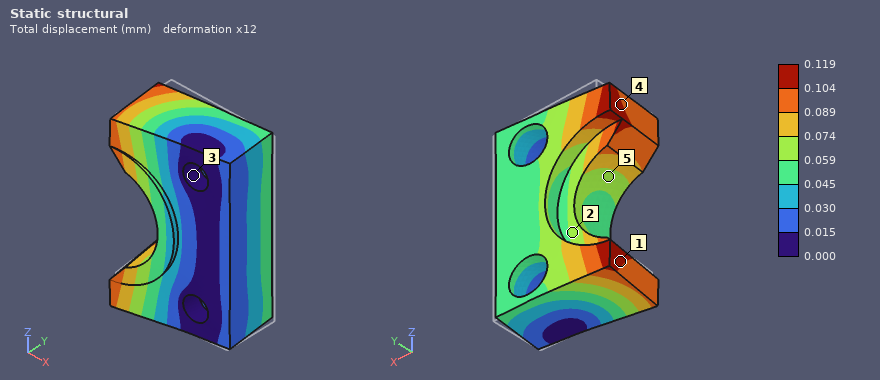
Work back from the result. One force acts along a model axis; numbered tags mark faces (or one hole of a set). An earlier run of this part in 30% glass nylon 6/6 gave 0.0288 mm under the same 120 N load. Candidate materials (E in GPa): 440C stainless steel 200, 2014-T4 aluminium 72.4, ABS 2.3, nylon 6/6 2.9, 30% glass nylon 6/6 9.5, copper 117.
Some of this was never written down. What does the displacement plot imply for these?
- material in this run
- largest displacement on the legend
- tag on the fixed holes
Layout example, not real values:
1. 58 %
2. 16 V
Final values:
1. ABS
2. 0.119 mm
3. 3
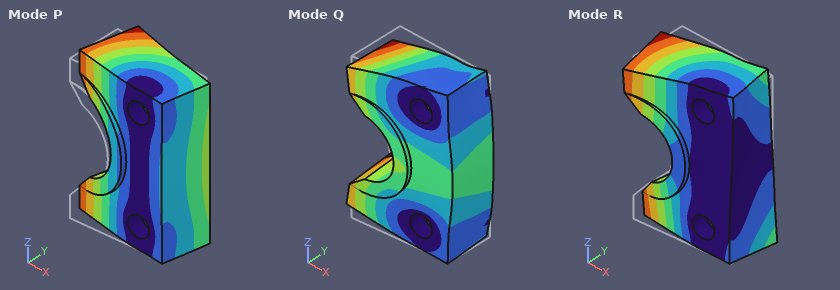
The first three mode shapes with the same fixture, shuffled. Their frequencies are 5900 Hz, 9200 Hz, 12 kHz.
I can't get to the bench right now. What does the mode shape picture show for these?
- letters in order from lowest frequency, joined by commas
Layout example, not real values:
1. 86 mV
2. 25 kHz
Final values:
1. P, R, Q
